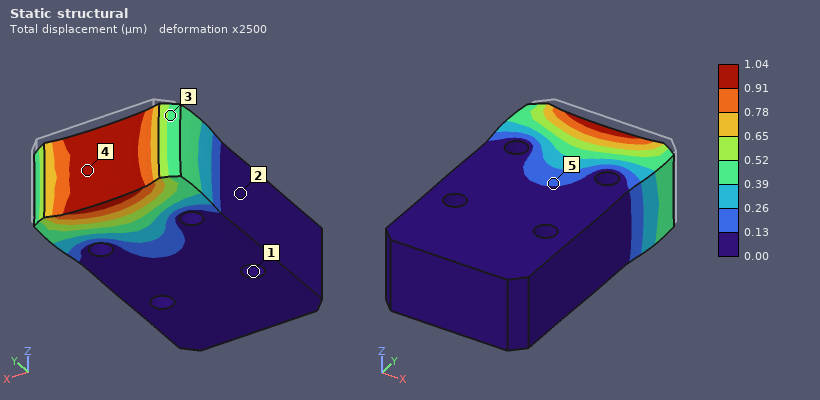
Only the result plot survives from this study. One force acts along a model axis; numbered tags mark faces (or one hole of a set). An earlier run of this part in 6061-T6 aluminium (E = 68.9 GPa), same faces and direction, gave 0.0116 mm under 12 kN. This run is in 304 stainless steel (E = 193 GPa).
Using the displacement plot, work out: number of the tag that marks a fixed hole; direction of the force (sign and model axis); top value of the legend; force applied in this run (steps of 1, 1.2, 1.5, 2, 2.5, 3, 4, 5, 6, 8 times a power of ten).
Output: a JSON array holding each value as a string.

["1", "-Y", "1.04 µm", "3 kN"]
